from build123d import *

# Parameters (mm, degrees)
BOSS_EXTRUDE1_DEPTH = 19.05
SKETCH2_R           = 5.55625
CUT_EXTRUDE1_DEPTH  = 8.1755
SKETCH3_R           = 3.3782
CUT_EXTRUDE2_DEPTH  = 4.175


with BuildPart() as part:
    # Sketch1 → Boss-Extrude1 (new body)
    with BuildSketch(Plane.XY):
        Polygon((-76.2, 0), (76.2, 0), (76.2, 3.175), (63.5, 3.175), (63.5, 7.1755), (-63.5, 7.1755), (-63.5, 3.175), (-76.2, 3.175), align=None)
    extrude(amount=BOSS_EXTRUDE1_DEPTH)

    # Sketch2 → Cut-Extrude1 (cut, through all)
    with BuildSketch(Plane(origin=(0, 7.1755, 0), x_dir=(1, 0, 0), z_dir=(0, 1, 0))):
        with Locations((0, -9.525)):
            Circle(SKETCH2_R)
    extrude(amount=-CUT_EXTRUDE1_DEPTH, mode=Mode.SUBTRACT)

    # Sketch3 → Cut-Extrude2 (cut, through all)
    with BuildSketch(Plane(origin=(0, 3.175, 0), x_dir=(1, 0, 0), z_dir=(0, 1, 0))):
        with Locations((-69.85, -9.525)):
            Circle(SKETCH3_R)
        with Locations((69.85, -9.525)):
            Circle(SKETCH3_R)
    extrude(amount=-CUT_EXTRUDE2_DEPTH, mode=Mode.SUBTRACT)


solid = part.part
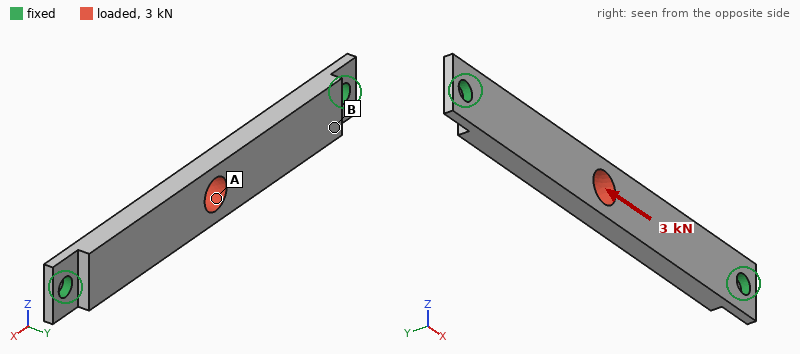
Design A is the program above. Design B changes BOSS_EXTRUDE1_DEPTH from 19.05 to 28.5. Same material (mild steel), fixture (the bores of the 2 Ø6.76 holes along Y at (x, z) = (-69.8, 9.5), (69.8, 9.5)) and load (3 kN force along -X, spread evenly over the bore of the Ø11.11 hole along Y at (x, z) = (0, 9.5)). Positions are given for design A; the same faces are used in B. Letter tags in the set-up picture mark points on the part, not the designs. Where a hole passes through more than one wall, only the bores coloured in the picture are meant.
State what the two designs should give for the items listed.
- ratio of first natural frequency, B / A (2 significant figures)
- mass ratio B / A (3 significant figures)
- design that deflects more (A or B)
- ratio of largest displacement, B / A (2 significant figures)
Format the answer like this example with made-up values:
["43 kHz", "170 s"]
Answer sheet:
["0.95", "1.52", "A", "0.87"]
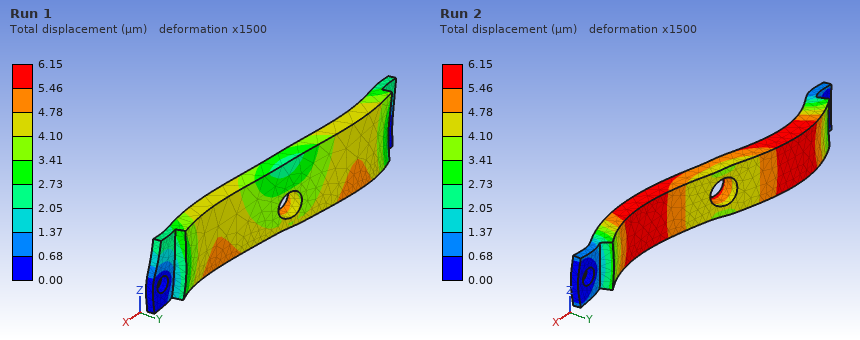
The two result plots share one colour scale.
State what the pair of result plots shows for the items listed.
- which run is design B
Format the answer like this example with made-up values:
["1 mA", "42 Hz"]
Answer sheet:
["Run 1"]
